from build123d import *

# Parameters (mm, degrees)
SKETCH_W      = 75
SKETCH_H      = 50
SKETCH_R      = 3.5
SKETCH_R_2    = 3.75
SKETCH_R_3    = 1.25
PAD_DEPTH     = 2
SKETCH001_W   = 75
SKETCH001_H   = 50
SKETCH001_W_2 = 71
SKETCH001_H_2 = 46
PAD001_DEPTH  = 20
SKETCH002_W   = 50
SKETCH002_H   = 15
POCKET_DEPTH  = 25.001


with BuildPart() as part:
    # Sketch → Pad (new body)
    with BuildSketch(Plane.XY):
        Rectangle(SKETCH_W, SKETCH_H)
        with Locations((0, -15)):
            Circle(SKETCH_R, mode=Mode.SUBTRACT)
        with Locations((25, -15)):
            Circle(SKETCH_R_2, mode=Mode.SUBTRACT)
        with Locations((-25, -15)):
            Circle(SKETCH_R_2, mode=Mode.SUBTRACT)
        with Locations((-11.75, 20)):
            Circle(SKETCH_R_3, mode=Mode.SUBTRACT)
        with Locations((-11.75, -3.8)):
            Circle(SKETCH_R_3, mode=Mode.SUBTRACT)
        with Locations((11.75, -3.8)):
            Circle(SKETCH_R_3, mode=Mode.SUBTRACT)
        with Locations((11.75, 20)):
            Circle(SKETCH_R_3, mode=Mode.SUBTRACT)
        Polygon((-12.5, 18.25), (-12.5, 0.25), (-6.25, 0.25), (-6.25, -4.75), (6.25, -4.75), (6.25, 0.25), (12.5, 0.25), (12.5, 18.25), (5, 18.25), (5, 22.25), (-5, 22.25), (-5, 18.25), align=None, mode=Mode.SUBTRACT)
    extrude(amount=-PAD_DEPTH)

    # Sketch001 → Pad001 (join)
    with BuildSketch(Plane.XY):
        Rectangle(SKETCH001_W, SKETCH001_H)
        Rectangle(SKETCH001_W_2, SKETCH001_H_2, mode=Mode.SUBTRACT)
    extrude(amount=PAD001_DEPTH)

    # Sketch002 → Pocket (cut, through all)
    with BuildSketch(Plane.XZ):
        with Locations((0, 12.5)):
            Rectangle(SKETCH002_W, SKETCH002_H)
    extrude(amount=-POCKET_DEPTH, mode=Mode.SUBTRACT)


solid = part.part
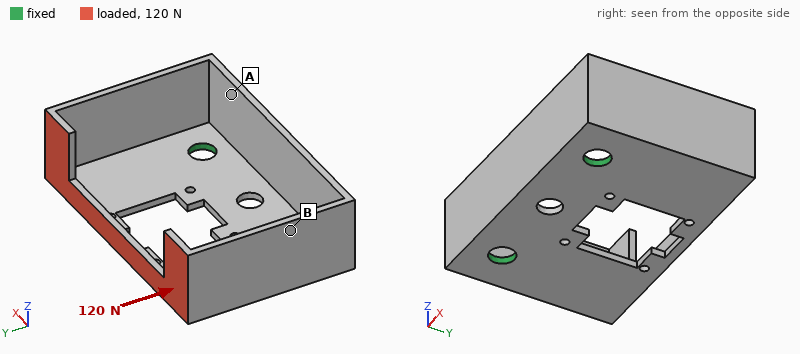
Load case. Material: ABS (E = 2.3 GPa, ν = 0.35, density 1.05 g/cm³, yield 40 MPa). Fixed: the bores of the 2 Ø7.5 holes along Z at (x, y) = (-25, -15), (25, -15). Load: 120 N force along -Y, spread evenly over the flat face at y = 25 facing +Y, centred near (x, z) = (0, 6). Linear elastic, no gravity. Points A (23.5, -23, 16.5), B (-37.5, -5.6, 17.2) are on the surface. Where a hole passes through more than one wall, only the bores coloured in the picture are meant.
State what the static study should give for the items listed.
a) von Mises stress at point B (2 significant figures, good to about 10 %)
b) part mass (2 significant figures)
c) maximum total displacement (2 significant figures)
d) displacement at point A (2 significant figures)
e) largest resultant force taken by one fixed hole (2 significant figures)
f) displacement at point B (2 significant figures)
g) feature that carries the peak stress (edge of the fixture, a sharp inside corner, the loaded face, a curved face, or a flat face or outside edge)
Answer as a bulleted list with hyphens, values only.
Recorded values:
- 2.4 MPa
- 15 g
- 1.0 mm
- 0.30 mm
- 60 N
- 0.41 mm
- a curved face
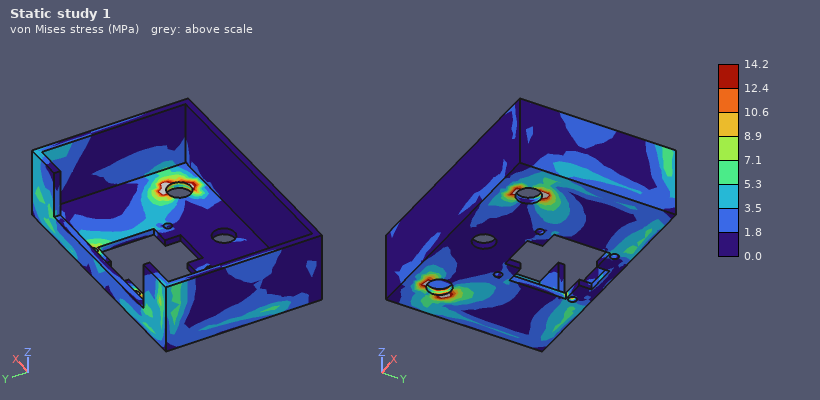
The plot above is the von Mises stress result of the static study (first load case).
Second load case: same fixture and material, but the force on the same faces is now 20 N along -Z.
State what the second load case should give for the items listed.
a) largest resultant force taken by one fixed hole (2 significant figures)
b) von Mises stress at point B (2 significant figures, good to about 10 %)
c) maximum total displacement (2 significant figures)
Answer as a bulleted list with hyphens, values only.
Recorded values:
- 10 N
- 2.2 MPa
- 0.90 mm
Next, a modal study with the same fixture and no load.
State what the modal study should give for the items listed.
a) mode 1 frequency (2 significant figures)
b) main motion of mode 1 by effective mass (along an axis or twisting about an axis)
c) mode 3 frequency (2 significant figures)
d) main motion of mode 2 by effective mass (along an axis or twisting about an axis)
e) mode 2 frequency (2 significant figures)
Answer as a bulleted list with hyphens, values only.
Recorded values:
- 380 Hz
- along Z
- 860 Hz
- twisting about Y
- 420 Hz
